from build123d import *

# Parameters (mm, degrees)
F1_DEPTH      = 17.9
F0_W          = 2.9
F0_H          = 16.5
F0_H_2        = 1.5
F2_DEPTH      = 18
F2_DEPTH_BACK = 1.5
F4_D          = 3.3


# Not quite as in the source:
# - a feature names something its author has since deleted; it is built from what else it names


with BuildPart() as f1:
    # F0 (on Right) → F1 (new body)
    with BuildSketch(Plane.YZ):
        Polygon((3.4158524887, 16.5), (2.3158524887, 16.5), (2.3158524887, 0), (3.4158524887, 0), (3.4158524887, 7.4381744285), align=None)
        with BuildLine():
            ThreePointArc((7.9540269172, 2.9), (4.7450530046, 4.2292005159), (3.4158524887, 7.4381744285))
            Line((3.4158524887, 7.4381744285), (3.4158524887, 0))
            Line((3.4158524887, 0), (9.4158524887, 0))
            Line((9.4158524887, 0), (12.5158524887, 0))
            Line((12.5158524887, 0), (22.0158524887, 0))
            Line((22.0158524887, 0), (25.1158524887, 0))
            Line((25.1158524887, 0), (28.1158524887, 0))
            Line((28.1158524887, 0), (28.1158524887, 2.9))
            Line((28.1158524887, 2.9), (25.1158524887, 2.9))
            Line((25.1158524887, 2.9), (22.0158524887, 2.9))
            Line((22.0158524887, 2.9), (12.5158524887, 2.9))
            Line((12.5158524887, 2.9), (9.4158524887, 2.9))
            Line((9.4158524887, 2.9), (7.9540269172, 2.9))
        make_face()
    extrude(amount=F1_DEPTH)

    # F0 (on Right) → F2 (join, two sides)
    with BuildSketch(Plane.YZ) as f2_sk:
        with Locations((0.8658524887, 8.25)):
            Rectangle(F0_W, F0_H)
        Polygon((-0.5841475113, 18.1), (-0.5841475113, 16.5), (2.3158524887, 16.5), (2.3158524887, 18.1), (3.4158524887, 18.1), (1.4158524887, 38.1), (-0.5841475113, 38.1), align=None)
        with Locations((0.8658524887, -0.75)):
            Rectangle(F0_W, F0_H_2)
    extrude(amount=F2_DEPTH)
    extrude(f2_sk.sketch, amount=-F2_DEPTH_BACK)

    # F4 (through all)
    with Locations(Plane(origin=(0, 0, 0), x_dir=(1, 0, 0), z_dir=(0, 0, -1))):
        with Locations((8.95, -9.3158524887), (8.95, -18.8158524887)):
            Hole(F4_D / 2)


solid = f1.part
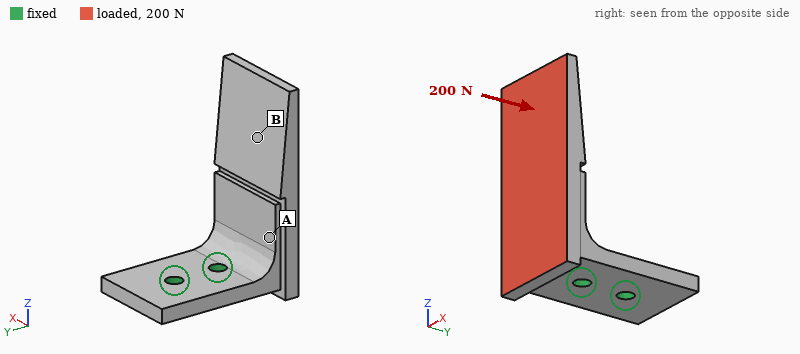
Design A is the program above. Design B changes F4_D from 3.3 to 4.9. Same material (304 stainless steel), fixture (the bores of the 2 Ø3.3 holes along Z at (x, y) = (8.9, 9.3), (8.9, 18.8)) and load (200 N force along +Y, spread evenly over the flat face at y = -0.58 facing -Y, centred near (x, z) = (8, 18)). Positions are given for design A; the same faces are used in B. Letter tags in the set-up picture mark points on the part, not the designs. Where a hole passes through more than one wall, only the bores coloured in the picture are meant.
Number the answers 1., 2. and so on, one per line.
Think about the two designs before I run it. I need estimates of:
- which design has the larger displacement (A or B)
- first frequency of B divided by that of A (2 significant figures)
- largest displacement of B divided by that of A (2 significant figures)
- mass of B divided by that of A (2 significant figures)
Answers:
1. A
2. 1.1
3. 0.85
4. 0.98
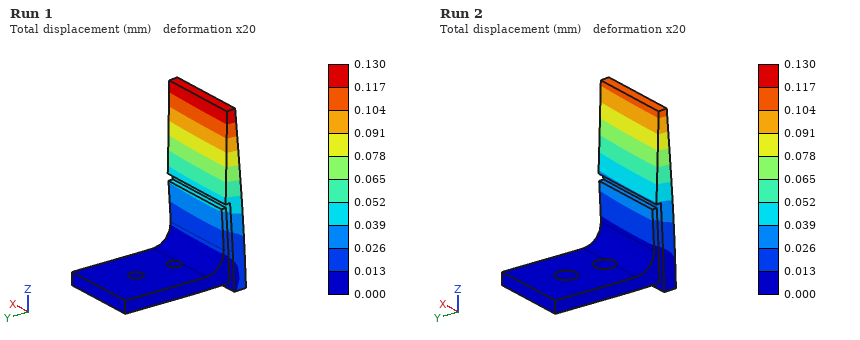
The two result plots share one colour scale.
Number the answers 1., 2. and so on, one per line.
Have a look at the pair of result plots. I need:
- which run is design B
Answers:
1. Run 2
